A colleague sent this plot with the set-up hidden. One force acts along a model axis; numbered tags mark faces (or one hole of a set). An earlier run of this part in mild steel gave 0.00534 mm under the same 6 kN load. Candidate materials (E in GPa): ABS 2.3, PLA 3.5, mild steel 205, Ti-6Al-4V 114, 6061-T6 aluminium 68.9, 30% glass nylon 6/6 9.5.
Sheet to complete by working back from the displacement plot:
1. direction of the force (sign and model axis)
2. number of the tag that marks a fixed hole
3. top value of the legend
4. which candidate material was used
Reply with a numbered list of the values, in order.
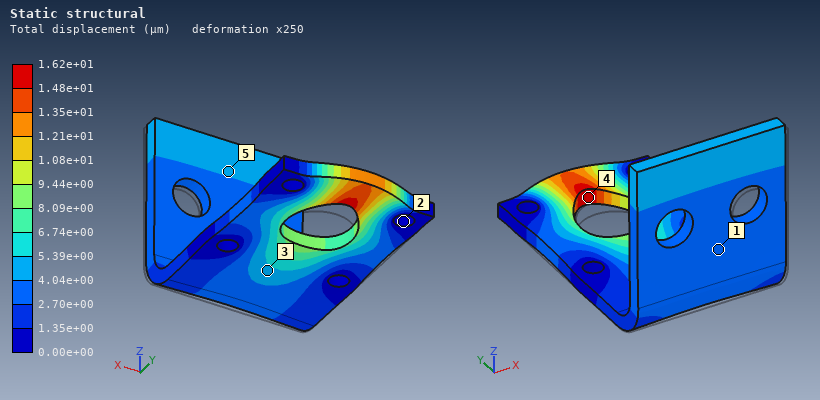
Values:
1. +Y
2. 2
3. 1.62e+01 µm
4. 6061-T6 aluminium
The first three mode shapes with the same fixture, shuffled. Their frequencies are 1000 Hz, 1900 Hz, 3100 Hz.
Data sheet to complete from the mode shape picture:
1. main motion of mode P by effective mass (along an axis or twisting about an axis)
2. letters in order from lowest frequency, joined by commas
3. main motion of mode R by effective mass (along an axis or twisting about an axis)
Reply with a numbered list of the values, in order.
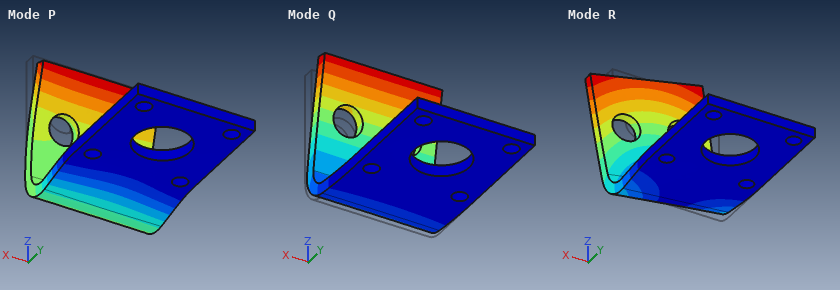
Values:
1. along Z
2. Q, R, P
3. along X
